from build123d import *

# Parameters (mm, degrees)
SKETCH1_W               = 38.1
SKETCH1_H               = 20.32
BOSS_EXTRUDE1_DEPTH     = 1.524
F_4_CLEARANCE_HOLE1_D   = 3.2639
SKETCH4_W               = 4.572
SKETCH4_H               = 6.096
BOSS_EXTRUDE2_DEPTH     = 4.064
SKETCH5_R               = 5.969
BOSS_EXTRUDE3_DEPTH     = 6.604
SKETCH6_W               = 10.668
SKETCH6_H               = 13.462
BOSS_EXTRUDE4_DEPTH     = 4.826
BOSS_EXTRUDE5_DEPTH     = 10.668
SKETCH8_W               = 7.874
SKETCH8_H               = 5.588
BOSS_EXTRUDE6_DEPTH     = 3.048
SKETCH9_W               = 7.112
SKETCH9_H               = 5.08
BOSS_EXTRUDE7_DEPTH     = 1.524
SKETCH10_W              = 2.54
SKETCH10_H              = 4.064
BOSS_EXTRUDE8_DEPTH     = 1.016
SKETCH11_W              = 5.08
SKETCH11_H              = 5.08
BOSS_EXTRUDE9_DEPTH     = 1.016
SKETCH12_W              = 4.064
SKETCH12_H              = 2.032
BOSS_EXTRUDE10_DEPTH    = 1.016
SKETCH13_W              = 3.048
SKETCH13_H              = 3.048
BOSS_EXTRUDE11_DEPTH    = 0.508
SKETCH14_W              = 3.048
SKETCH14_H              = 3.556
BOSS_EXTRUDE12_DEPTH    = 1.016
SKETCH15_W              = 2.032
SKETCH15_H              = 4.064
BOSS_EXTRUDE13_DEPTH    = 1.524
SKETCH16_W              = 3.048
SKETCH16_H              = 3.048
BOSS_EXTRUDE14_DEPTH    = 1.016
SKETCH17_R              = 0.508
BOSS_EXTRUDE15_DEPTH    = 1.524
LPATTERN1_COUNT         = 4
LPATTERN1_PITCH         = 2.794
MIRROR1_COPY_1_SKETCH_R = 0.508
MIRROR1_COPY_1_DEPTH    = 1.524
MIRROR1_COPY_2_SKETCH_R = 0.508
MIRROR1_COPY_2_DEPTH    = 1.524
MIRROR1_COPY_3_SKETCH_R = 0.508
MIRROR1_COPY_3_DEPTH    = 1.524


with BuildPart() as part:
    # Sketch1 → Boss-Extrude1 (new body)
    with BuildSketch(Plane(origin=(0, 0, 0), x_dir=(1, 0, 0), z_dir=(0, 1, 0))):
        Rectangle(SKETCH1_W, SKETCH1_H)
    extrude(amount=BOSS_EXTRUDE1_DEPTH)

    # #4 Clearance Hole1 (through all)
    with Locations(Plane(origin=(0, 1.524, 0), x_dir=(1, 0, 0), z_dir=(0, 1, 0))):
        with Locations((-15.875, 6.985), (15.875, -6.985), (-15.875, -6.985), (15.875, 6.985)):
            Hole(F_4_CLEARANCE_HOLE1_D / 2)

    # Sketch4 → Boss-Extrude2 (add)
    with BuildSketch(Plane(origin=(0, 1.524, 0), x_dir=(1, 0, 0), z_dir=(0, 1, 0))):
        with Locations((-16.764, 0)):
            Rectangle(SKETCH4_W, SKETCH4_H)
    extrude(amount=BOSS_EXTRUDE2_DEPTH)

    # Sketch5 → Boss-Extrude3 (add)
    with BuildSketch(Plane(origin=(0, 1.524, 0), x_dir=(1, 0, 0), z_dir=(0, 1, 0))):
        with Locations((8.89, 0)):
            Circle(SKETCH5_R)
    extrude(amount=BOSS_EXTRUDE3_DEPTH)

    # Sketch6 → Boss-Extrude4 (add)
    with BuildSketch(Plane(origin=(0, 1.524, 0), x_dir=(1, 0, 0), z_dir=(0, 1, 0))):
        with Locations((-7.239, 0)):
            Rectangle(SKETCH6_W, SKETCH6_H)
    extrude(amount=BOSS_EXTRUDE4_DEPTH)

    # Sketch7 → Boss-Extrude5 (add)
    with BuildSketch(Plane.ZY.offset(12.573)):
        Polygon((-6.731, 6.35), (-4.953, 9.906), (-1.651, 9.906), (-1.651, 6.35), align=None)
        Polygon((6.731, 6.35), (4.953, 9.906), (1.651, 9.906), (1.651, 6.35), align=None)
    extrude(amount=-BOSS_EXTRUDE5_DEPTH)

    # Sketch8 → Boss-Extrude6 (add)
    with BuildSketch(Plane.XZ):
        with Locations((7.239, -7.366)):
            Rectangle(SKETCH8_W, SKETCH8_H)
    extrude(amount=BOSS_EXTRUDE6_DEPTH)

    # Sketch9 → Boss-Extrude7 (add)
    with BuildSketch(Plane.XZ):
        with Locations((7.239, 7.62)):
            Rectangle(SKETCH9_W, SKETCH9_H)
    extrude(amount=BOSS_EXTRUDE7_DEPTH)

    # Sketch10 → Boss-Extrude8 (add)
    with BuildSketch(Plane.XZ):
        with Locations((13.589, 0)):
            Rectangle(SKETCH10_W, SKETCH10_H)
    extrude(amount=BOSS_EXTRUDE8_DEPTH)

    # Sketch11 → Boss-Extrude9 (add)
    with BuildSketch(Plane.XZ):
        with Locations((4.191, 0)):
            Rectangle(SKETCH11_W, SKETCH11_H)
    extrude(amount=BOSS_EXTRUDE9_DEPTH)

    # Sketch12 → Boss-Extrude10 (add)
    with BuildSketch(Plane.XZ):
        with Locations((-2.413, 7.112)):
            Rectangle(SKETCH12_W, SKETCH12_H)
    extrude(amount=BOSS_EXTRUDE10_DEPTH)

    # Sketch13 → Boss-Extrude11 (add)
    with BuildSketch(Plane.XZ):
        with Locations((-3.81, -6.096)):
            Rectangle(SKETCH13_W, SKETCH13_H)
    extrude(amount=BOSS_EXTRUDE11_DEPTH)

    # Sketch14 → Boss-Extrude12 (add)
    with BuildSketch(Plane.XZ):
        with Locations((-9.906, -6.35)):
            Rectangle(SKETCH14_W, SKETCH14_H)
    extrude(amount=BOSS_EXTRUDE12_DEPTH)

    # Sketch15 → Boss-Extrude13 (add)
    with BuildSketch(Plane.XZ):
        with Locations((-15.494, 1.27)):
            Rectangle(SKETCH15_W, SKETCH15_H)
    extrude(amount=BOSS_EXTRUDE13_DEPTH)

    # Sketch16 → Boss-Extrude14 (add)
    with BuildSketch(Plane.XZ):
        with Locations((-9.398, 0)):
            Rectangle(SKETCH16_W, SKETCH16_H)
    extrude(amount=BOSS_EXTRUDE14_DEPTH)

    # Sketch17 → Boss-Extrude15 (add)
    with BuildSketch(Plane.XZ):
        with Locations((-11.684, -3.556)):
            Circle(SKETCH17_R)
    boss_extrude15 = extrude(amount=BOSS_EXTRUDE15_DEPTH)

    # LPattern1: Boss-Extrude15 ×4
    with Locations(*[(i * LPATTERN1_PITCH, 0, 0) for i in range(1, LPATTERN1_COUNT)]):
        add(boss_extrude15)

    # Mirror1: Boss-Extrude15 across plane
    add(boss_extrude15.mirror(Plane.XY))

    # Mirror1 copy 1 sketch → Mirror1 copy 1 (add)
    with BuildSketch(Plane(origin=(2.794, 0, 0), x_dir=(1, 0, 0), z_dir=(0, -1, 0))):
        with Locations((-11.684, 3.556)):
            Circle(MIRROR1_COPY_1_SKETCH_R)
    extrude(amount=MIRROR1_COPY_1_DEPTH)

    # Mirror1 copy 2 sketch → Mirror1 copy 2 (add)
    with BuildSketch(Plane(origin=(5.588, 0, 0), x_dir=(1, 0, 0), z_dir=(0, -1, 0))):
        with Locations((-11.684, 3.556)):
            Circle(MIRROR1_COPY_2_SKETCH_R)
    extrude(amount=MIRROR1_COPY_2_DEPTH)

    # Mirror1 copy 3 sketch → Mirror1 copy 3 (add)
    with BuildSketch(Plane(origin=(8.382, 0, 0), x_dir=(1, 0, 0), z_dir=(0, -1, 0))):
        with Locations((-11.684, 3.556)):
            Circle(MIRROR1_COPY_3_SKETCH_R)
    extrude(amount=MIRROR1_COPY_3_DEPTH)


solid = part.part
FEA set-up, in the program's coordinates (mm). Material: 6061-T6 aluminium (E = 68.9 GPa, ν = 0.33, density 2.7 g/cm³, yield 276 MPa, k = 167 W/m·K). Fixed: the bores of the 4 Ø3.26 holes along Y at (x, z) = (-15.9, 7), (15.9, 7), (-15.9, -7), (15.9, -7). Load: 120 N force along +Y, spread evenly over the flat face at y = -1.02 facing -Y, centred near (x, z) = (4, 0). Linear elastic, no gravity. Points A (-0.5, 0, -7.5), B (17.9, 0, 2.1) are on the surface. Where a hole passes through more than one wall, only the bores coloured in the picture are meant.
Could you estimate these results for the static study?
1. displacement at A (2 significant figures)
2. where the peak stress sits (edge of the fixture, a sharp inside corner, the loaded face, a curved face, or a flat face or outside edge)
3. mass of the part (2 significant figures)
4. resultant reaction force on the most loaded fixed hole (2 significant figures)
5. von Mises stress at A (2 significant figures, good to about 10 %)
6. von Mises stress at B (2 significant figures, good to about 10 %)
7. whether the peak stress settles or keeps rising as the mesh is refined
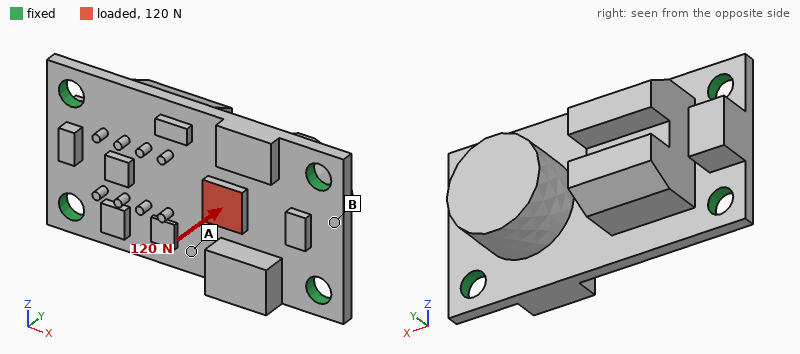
23 µm
edge of the fixture
8.8 g
44 N
26 MPa
10 MPa
keeps rising
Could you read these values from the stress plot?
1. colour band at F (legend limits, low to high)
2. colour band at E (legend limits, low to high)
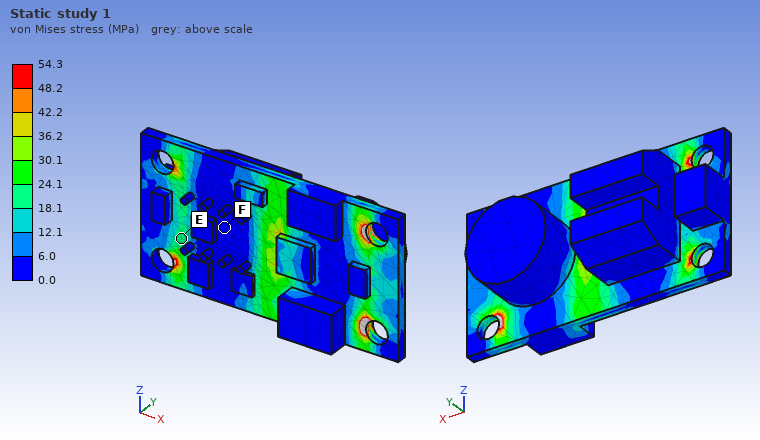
0.0 to 6.0 MPa
18.1 to 24.1 MPa
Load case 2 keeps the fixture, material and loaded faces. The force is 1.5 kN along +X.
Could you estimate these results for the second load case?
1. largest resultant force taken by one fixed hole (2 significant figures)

480 N
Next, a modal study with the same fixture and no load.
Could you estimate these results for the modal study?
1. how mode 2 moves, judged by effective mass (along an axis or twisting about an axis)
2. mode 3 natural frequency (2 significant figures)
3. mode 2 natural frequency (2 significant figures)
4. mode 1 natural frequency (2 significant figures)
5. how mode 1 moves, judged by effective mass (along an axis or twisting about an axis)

along Z
23 kHz
17 kHz
5600 Hz
along Y
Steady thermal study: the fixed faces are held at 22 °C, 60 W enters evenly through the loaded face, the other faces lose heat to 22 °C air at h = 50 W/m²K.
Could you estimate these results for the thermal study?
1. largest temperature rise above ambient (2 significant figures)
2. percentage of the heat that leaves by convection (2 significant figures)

84 K
5.5 %
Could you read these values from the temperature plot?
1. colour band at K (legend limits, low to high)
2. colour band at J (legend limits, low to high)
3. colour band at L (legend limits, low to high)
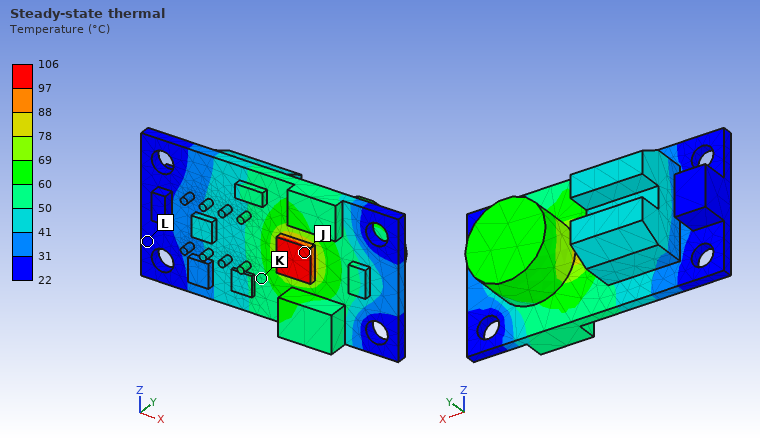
50 to 60 °C
97 to 106 °C
22 to 31 °C
